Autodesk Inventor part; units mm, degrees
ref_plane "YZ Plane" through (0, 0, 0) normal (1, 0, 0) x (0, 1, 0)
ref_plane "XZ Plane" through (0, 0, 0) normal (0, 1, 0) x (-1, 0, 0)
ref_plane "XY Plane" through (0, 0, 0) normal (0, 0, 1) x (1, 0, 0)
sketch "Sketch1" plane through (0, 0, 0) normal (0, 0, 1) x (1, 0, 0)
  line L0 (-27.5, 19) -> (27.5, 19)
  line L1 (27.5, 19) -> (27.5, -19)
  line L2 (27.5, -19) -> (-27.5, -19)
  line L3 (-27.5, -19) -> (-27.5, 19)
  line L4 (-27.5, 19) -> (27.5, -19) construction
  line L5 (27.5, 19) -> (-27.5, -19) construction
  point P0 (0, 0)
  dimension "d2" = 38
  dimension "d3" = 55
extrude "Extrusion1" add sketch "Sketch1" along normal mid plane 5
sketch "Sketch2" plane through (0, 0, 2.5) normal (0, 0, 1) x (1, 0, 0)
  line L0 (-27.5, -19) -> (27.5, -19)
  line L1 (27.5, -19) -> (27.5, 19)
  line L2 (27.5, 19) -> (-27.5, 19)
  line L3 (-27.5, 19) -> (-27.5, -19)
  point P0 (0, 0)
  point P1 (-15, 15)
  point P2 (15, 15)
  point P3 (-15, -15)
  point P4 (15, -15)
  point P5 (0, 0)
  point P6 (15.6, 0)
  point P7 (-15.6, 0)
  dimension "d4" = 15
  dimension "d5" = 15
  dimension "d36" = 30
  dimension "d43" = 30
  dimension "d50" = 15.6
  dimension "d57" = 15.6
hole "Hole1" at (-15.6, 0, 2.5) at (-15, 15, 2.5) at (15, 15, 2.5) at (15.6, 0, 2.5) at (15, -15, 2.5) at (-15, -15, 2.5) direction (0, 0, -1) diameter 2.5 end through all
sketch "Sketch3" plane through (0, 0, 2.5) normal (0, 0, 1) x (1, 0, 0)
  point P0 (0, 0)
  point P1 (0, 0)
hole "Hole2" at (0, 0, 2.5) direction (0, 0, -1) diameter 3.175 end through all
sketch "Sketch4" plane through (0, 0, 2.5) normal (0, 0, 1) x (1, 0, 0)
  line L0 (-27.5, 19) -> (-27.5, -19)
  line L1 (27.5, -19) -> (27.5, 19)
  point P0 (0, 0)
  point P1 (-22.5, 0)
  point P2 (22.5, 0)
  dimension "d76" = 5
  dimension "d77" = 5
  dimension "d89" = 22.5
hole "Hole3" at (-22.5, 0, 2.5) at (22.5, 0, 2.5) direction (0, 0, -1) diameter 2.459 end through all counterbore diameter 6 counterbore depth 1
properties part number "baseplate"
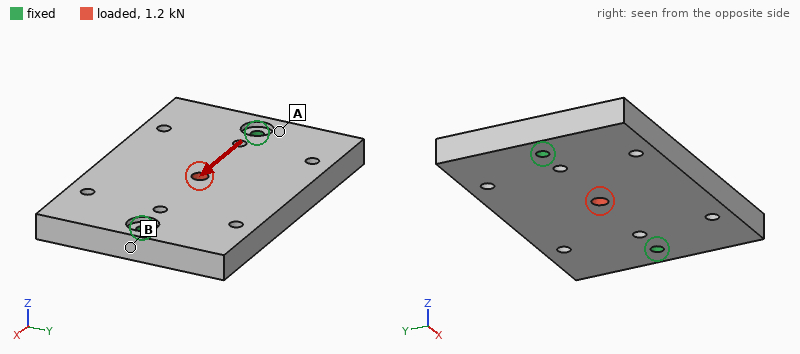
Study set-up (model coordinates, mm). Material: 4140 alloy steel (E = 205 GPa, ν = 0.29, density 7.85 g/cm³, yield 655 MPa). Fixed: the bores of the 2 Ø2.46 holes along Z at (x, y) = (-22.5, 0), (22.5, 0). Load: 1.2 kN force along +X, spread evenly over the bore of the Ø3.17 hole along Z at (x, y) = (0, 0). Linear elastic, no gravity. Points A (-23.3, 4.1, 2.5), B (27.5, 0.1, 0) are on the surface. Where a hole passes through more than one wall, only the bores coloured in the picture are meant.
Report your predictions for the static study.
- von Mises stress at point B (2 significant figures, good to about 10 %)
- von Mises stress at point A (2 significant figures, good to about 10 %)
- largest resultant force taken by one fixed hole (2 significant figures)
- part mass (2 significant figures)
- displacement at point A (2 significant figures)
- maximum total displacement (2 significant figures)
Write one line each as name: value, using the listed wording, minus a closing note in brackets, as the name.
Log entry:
von Mises stress at point B: 11 MPa
von Mises stress at point A: 4.9 MPa
largest resultant force taken by one fixed hole: 600 N
part mass: 80 g
displacement at point A: 0.36 µm
maximum total displacement: 1.4 µm
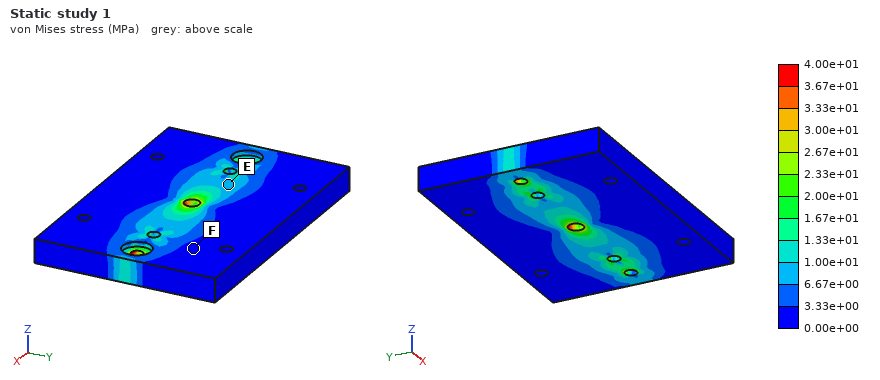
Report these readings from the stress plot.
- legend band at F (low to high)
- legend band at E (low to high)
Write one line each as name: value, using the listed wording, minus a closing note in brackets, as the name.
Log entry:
legend band at F: 0.00e+00 to 3.33e+00 MPa
legend band at E: 6.67e+00 to 1.00e+01 MPa
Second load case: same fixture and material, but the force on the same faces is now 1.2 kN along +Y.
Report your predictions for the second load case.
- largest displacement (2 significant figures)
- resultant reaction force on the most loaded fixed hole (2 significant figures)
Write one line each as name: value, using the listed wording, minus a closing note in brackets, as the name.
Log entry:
largest displacement: 2.3 µm
resultant reaction force on the most loaded fixed hole: 600 N
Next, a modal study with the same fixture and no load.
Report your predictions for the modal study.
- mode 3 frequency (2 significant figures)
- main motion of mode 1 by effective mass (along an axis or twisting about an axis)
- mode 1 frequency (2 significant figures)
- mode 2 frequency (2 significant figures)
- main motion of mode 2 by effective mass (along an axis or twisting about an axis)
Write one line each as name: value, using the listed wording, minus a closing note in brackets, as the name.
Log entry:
mode 3 frequency: 10 kHz
main motion of mode 1 by effective mass: twisting about X
mode 1 frequency: 4900 Hz
mode 2 frequency: 6800 Hz
main motion of mode 2 by effective mass: along Z
